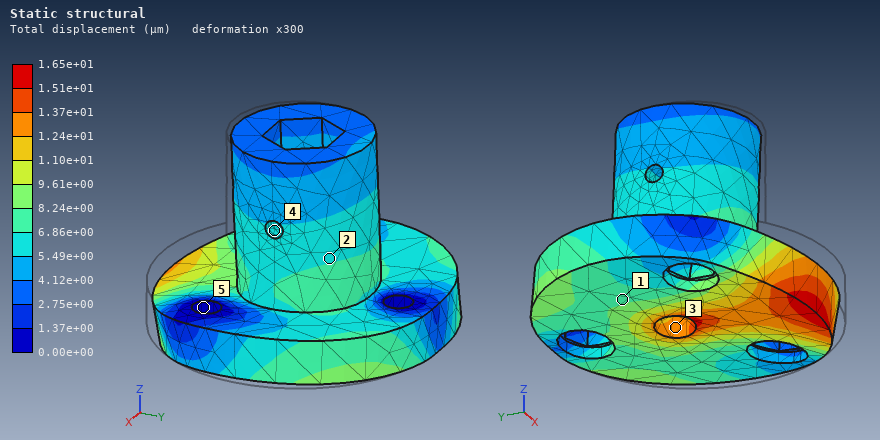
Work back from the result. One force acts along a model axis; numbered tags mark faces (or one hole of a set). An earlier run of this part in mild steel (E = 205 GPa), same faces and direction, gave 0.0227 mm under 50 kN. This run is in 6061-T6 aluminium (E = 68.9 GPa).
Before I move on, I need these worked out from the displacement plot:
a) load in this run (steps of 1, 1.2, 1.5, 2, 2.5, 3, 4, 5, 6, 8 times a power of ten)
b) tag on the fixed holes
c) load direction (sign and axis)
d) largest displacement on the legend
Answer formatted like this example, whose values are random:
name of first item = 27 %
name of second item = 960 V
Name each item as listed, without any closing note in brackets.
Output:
load in this run = 12 kN
tag on the fixed holes = 5
load direction = +Y
largest displacement on the legend = 1.65e+01 µm
